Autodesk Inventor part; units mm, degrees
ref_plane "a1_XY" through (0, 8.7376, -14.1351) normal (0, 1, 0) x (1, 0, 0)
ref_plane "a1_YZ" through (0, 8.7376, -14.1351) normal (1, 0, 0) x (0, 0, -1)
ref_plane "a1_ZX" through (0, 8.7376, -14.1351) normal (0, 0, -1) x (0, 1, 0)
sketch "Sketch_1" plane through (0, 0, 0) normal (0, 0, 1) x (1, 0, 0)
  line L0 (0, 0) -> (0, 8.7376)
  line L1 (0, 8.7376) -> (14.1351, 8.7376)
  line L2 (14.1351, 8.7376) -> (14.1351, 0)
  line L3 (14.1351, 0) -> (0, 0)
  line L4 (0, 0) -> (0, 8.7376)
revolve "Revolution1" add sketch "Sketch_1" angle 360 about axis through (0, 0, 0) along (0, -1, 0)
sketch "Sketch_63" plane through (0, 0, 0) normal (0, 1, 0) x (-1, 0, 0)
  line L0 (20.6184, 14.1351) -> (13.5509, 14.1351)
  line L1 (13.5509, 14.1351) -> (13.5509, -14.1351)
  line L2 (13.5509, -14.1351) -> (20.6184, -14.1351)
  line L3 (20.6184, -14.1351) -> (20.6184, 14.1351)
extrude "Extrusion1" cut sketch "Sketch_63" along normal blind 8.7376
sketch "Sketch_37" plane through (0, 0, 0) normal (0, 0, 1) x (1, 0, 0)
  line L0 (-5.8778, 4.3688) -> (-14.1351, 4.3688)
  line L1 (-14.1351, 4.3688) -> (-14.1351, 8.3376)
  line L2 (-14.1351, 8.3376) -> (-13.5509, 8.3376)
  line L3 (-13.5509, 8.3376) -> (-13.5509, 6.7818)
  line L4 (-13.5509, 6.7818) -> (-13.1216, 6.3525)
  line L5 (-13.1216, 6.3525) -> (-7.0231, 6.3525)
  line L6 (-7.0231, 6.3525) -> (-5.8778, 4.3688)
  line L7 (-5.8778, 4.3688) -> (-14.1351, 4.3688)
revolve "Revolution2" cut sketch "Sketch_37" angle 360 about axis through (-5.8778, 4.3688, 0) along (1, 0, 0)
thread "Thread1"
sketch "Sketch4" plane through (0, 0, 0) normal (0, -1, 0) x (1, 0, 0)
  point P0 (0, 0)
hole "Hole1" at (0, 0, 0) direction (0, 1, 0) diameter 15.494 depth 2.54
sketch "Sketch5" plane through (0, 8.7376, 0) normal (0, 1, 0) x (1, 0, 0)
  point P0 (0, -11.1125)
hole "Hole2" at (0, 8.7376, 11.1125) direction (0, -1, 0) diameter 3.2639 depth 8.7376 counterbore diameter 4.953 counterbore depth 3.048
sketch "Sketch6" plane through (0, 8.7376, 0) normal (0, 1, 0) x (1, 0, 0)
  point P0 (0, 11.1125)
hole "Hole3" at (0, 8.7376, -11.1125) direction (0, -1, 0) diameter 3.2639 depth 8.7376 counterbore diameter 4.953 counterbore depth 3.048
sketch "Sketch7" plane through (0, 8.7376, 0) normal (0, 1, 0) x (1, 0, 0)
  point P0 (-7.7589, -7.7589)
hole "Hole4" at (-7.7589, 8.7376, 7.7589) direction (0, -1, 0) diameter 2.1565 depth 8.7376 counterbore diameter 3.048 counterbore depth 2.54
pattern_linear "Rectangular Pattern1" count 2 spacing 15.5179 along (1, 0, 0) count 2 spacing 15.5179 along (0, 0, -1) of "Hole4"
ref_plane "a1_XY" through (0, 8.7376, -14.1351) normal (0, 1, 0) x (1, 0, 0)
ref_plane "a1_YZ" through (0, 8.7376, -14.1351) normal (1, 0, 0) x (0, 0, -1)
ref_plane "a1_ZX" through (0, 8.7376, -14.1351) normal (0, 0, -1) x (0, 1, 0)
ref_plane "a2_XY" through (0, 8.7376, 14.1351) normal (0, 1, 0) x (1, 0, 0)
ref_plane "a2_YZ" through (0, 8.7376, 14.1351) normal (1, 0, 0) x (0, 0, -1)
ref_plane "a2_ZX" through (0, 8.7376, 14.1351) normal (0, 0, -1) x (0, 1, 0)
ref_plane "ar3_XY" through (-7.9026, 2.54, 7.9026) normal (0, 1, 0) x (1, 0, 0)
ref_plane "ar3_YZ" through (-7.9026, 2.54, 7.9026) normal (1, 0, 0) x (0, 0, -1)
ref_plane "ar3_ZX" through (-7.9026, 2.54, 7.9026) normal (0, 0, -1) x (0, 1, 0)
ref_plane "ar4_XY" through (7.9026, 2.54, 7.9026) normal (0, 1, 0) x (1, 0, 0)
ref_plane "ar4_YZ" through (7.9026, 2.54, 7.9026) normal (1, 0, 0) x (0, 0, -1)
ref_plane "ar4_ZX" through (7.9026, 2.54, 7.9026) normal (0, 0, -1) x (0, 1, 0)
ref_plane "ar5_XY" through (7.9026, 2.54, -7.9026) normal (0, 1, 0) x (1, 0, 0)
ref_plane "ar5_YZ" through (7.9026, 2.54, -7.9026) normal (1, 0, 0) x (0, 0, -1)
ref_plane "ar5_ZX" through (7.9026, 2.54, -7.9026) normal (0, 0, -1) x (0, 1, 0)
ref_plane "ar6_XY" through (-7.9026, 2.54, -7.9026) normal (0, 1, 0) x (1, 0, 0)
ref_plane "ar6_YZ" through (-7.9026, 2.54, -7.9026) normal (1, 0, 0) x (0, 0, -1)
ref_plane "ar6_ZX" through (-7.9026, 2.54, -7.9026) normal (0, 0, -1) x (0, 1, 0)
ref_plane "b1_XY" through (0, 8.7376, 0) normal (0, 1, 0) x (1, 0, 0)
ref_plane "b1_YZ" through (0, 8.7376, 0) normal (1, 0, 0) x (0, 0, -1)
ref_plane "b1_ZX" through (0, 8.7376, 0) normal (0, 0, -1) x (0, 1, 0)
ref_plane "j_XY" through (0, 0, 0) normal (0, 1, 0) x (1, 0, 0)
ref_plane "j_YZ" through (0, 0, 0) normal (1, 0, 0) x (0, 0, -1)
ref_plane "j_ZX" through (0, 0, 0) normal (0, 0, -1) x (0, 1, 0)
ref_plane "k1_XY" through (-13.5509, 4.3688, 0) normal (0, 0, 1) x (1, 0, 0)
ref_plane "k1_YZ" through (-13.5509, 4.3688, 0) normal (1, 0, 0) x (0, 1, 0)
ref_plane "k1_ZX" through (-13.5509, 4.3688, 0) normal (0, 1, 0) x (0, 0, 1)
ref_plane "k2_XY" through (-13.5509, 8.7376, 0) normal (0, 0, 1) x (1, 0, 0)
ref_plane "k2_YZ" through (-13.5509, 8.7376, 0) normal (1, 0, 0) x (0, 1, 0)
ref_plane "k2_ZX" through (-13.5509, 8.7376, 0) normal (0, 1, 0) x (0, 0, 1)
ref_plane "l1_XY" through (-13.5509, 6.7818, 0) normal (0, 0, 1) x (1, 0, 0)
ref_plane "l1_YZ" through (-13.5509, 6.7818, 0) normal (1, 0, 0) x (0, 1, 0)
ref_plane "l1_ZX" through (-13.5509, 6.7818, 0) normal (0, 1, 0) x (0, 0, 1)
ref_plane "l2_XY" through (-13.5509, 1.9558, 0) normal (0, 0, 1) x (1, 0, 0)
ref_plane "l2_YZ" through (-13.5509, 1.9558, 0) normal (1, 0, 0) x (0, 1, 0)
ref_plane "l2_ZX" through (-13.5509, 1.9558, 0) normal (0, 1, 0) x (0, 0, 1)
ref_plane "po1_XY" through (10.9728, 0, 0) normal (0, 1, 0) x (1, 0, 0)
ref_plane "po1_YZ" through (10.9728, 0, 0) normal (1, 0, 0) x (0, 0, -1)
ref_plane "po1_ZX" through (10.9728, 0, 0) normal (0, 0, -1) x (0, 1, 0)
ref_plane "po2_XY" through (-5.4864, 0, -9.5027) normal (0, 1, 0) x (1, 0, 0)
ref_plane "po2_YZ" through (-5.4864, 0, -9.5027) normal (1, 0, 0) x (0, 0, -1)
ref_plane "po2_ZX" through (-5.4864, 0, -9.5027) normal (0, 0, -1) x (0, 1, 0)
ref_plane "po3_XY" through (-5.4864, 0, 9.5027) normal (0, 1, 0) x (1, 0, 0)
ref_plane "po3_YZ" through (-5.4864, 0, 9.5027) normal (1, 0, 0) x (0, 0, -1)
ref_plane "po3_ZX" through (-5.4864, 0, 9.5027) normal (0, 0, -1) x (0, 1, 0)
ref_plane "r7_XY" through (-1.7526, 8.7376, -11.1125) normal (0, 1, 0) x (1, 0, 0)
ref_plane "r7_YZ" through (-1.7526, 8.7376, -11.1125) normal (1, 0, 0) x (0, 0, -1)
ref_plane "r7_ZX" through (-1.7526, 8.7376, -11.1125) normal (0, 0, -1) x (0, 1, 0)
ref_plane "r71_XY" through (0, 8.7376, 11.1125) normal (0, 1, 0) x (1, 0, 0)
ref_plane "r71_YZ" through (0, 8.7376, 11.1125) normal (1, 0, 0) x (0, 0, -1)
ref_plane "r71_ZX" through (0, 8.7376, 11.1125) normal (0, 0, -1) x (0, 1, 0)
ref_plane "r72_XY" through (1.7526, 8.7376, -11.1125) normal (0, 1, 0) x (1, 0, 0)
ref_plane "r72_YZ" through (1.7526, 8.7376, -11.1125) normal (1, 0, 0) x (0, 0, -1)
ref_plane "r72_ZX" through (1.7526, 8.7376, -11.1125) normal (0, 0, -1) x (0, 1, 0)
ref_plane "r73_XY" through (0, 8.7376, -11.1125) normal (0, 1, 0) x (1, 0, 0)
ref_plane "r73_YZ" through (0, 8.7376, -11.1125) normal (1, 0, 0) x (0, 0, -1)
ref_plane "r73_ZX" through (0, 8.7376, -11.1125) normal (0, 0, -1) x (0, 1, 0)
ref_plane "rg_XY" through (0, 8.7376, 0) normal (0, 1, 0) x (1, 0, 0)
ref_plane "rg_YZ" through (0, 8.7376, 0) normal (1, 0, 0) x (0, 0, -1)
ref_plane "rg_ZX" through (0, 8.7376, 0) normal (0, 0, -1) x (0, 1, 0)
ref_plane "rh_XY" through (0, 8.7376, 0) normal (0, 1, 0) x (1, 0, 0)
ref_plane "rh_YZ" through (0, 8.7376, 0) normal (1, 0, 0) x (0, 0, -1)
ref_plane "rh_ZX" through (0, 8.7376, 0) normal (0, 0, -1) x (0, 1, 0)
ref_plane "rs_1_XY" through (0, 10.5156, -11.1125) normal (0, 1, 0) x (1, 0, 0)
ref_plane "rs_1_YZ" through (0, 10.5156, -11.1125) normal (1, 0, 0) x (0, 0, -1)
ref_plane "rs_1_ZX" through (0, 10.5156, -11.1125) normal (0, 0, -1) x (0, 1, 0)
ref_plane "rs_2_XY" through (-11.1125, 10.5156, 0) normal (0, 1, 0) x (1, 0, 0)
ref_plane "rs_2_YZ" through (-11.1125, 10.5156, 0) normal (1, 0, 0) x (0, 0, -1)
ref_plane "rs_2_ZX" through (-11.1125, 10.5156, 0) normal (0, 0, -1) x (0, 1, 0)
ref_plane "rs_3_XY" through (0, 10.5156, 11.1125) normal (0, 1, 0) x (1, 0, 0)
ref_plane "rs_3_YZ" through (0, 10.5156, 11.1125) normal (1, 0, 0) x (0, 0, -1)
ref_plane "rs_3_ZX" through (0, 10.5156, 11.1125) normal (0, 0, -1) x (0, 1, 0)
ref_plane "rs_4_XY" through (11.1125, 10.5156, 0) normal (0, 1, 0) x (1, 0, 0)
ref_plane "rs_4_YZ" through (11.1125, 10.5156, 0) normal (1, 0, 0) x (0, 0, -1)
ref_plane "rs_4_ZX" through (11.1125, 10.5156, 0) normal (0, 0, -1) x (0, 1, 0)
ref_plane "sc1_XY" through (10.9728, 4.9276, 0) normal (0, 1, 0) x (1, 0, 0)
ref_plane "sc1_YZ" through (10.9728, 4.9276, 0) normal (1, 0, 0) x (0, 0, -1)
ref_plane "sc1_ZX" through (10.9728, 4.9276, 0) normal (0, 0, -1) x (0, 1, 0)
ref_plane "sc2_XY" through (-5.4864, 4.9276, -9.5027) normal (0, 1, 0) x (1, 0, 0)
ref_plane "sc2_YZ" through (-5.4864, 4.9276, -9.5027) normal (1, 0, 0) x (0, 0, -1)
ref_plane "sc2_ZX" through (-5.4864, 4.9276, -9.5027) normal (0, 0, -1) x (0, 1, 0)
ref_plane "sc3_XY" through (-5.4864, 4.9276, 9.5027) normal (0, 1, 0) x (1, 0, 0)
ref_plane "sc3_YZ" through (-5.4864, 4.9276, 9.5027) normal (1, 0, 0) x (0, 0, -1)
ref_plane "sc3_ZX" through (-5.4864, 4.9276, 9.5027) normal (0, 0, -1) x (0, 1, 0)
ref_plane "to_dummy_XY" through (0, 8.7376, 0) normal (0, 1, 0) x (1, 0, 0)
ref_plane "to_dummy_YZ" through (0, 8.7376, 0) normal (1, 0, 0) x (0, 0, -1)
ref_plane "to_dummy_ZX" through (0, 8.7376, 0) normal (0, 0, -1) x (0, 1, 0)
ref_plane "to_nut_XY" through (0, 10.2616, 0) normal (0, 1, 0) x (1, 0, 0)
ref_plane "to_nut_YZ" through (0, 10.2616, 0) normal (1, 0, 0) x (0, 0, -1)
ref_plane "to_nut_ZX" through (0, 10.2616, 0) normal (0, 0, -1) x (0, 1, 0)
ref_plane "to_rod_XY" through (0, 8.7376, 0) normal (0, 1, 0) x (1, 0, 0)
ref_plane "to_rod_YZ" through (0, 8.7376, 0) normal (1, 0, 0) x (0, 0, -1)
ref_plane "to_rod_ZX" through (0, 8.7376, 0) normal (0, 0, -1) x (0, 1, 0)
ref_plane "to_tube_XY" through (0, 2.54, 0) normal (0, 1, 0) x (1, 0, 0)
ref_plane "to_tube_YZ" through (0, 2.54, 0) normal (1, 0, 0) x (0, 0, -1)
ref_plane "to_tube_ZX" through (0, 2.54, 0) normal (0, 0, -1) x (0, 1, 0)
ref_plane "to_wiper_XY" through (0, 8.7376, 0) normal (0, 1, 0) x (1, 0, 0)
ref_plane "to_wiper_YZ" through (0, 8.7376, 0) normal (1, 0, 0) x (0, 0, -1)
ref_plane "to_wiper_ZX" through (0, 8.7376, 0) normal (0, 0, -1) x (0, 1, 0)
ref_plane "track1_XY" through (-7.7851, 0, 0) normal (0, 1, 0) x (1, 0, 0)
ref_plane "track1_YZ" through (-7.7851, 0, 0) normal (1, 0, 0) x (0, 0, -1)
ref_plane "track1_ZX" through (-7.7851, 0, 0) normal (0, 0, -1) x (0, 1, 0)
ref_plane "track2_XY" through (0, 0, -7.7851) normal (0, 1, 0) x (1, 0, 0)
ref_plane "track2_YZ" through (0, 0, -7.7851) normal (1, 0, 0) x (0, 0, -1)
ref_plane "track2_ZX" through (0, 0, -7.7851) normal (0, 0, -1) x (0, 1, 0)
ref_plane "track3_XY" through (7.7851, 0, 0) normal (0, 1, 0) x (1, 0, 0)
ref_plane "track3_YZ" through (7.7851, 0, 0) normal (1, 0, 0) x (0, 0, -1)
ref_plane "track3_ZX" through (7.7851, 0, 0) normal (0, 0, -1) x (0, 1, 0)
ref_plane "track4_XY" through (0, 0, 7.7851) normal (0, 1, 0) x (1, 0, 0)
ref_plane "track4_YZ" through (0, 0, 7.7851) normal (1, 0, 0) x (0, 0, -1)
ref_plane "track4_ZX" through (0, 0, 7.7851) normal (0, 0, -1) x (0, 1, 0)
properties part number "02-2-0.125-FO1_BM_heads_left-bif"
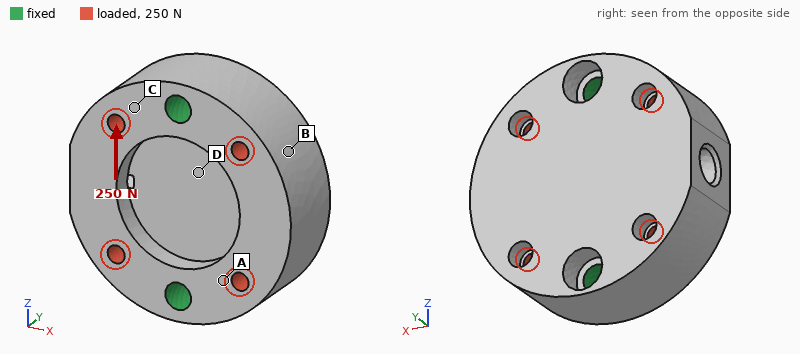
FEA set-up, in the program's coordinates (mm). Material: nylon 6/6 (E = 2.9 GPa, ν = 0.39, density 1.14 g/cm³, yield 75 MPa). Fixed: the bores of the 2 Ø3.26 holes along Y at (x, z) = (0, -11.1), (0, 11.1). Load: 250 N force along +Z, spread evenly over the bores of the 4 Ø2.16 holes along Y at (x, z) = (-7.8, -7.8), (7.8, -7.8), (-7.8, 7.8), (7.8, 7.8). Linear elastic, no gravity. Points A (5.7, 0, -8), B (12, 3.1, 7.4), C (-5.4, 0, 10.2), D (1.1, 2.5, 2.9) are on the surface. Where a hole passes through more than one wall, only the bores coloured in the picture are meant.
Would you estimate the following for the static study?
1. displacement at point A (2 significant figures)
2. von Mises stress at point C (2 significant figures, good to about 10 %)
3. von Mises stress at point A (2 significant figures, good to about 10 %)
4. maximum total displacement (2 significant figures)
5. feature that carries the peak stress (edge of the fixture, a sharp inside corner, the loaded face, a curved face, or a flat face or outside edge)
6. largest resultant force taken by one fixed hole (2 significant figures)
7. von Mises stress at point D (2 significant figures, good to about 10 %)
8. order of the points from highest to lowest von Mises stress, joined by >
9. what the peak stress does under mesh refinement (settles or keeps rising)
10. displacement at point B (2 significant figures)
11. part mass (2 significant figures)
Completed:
8.2 µm
1.9 MPa
2.2 MPa
13 µm
edge of the fixture
130 N
1.1 MPa
A > C > D > B
keeps rising
9.6 µm
5.1 g
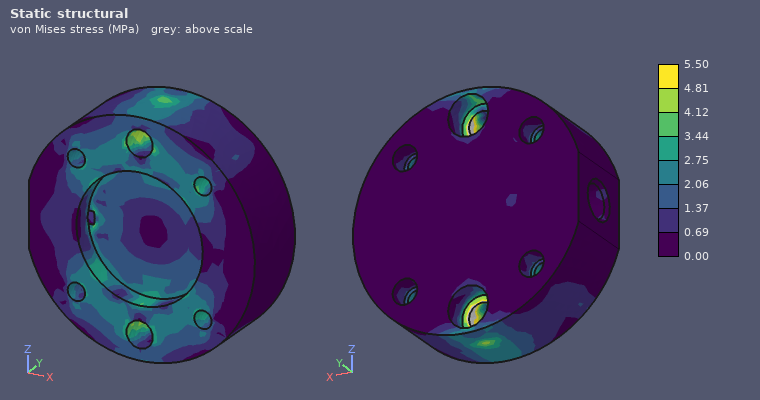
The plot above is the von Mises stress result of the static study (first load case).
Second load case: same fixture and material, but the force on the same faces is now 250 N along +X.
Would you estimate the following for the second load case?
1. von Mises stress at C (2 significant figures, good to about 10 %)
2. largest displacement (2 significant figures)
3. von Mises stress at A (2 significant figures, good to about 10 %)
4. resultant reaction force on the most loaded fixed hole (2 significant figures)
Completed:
1.9 MPa
7.3 µm
2.1 MPa
130 N
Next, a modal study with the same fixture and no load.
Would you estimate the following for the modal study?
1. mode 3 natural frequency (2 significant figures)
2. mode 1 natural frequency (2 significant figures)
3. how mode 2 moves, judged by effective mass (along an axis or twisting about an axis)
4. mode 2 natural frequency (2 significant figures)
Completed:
13 kHz
5600 Hz
along Y
8200 Hz
